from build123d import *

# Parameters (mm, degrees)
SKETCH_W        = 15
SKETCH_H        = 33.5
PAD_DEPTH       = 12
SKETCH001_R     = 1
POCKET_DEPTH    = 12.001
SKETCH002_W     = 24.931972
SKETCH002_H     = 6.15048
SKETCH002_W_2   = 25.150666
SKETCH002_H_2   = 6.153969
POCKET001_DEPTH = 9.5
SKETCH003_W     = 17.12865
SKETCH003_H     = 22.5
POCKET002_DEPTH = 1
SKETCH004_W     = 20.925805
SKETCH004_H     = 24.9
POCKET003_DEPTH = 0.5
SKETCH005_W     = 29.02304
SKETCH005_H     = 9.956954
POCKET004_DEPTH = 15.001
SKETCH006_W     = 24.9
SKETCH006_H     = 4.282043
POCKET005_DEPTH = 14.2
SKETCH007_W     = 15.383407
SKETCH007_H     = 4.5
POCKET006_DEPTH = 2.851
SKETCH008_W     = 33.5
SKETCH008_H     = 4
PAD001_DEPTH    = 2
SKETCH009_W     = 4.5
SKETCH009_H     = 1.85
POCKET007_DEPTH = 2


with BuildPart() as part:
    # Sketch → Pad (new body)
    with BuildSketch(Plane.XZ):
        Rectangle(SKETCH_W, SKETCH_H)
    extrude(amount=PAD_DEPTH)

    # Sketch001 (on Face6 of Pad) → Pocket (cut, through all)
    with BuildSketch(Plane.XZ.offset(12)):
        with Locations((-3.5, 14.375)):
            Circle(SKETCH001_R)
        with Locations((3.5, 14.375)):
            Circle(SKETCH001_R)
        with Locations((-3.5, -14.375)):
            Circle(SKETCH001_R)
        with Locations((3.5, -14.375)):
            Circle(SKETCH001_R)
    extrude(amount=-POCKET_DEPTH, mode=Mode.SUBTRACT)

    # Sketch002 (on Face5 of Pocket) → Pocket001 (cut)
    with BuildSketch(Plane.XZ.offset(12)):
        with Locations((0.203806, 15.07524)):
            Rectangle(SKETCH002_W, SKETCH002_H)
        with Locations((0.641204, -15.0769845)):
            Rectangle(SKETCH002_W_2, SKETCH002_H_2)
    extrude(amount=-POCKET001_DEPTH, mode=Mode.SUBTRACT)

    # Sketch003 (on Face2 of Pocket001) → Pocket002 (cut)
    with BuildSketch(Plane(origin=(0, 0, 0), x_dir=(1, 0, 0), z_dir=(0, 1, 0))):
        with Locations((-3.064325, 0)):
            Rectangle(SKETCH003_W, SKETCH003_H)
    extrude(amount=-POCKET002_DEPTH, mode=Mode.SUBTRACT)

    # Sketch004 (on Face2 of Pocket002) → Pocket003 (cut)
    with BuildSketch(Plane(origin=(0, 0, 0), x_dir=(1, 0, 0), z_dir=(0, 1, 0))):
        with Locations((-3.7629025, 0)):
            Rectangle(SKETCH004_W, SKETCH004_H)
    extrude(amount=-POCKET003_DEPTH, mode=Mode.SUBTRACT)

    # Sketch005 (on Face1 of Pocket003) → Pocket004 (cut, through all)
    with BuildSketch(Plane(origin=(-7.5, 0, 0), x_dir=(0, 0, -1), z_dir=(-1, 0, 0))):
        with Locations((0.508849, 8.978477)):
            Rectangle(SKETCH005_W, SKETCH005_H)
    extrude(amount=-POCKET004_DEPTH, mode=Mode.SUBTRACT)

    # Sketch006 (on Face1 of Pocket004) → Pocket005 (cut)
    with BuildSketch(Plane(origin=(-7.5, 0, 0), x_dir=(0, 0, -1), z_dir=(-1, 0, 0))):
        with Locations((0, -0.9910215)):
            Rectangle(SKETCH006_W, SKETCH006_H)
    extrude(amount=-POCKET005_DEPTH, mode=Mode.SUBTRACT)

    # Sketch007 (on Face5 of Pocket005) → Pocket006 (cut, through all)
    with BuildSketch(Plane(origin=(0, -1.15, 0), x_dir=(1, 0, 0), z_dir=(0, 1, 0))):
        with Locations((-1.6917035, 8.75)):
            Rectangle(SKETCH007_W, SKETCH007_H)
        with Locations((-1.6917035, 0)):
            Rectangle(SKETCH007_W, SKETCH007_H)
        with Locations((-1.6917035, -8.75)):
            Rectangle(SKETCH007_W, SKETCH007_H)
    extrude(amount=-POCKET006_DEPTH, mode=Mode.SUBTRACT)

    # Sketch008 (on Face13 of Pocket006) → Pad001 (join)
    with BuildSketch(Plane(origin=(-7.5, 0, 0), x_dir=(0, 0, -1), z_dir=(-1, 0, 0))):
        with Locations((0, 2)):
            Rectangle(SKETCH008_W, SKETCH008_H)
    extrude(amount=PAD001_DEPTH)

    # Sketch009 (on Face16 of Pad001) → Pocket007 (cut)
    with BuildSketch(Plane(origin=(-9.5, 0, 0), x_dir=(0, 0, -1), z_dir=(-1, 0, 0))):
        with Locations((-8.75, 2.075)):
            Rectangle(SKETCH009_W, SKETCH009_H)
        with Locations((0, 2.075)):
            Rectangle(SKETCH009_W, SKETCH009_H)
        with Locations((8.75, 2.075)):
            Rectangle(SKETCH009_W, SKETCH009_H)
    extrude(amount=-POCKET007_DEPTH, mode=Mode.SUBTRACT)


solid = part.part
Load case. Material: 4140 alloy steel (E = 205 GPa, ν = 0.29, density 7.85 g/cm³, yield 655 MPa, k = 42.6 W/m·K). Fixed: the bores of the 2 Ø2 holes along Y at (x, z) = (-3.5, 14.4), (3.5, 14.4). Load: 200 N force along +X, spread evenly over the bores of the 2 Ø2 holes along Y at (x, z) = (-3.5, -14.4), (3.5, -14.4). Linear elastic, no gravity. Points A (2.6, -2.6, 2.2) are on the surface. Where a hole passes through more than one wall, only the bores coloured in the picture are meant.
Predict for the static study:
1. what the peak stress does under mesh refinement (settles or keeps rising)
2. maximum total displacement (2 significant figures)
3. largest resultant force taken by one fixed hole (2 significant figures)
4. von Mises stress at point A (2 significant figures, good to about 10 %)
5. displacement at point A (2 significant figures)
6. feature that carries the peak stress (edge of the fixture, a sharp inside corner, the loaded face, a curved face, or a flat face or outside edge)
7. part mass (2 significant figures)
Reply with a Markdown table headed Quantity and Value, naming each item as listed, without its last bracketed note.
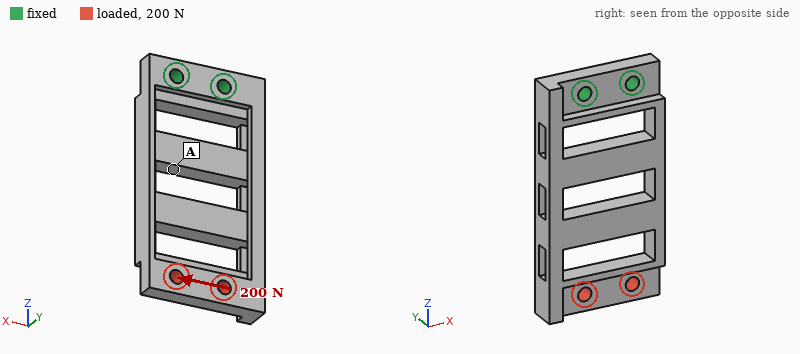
| Quantity | Value |
|---|---|
| what the peak stress does under mesh refinement | keeps rising |
| maximum total displacement | 92 µm |
| largest resultant force taken by one fixed hole | 510 N |
| von Mises stress at point A | 53 MPa |
| displacement at point A | 27 µm |
| feature that carries the peak stress | a sharp inside corner |
| part mass | 8.3 g |
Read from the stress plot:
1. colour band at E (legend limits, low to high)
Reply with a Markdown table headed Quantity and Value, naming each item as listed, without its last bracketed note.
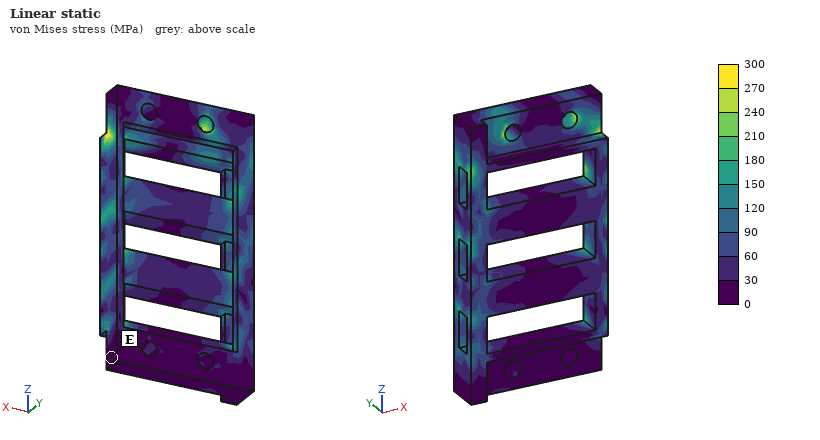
| Quantity | Value |
|---|---|
| colour band at E | 0 to 30 MPa |
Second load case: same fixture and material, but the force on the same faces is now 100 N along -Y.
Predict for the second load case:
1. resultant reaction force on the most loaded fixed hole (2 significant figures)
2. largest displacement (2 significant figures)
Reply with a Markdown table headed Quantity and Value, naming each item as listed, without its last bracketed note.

| Quantity | Value |
|---|---|
| resultant reaction force on the most loaded fixed hole | 66 N |
| largest displacement | 0.40 mm |
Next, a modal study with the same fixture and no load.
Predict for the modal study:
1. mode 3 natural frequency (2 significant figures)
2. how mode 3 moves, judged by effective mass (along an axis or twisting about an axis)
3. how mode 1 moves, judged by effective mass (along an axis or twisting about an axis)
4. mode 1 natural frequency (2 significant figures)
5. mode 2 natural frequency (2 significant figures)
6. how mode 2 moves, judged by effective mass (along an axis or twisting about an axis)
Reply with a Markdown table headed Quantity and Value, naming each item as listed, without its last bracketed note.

| Quantity | Value |
|---|---|
| mode 3 natural frequency | 5600 Hz |
| how mode 3 moves, judged by effective mass | along X |
| how mode 1 moves, judged by effective mass | along Y |
| mode 1 natural frequency | 1600 Hz |
| mode 2 natural frequency | 4400 Hz |
| how mode 2 moves, judged by effective mass | along X |
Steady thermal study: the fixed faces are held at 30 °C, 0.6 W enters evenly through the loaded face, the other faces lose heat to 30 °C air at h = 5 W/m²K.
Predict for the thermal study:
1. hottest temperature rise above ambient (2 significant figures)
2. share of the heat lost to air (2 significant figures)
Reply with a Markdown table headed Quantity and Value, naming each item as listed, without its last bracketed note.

| Quantity | Value |
|---|---|
| hottest temperature rise above ambient | 31 K |
| share of the heat lost to air | 19 % |
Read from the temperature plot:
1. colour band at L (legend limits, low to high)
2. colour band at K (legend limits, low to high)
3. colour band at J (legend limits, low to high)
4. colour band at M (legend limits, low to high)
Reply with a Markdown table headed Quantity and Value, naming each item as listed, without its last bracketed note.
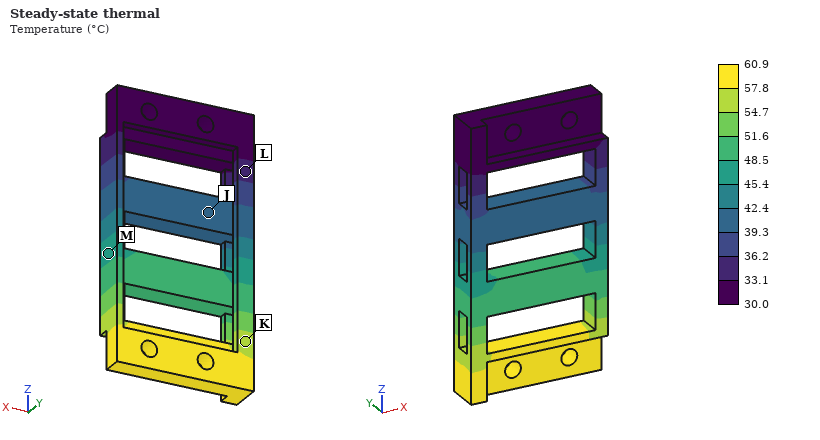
| Quantity | Value |
|---|---|
| colour band at L | 33.1 to 36.2 °C |
| colour band at K | 54.7 to 57.8 °C |
| colour band at J | 39.3 to 42.4 °C |
| colour band at M | 45.4 to 48.5 °C |
